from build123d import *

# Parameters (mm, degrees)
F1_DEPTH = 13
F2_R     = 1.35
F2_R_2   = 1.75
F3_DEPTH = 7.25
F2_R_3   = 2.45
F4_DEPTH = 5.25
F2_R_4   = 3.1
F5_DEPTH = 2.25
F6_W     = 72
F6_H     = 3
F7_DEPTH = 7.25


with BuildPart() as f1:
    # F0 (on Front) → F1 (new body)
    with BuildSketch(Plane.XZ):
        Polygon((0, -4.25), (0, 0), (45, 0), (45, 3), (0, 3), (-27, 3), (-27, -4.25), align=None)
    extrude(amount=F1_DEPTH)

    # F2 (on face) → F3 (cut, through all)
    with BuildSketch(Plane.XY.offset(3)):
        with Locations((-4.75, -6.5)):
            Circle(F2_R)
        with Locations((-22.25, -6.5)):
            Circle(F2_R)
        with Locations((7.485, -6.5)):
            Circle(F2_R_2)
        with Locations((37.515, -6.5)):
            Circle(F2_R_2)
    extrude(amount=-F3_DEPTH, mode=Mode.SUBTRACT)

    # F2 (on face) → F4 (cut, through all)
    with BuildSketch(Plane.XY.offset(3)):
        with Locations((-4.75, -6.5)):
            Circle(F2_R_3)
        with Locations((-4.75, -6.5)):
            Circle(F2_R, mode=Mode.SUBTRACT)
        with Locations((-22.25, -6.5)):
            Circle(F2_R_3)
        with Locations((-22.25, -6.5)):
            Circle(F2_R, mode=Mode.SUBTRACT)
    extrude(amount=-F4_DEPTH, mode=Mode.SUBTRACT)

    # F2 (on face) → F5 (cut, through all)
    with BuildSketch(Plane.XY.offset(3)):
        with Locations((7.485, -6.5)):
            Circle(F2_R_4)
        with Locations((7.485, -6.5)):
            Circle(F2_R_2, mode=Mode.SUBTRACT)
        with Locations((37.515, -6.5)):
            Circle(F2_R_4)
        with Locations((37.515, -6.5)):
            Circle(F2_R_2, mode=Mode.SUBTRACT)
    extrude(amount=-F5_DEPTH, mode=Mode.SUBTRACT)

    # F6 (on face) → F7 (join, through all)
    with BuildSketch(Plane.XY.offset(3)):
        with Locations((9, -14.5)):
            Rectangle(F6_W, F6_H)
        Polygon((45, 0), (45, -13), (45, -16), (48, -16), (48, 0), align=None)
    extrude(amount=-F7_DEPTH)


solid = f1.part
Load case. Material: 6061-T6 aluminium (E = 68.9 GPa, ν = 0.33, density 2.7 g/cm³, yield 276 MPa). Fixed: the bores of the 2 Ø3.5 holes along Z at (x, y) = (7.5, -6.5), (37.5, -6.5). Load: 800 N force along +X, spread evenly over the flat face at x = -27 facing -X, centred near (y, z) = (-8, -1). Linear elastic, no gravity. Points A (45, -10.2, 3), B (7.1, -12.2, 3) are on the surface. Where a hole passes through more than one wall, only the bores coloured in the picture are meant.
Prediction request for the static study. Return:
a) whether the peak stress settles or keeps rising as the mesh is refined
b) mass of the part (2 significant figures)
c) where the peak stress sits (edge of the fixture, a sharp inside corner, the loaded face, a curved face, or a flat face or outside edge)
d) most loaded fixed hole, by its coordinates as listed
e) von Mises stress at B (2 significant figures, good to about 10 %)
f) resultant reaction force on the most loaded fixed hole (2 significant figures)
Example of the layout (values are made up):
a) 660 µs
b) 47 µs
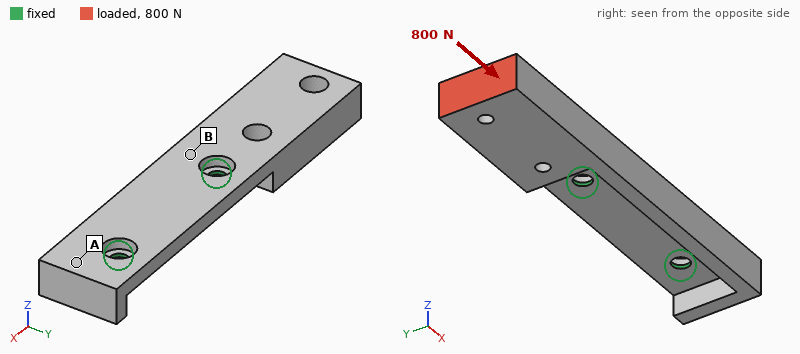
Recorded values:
a) keeps rising
b) 16 g
c) edge of the fixture
d) (7.5, -6.5)
e) 13 MPa
f) 630 N
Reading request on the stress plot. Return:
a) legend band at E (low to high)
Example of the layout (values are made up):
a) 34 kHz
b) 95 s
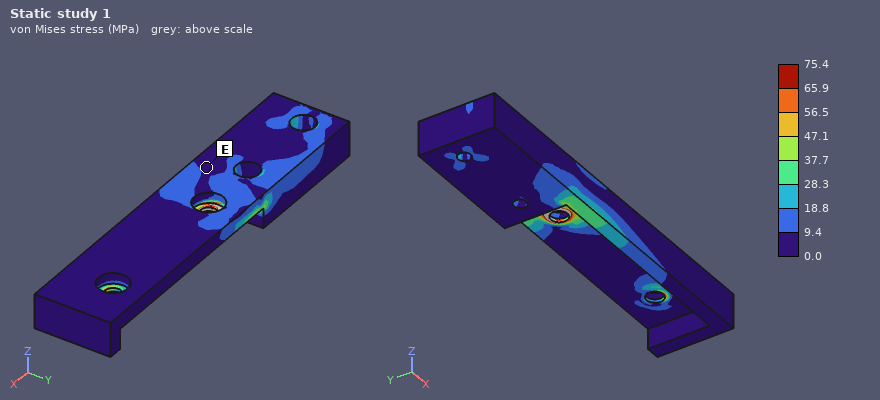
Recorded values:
a) 0.0 to 9.4 MPa
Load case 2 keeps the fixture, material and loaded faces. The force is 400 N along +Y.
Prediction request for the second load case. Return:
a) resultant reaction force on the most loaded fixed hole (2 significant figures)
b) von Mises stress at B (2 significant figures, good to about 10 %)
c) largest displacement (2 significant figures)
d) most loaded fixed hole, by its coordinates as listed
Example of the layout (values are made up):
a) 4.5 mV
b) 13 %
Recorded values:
a) 880 N
b) 59 MPa
c) 0.17 mm
d) (7.5, -6.5)
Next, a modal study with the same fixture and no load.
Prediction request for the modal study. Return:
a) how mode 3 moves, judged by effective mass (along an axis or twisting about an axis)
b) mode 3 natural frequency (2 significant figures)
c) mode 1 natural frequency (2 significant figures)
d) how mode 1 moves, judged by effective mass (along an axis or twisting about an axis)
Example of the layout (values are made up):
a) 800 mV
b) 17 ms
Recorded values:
a) along Y
b) 4900 Hz
c) 1800 Hz
d) along Z
